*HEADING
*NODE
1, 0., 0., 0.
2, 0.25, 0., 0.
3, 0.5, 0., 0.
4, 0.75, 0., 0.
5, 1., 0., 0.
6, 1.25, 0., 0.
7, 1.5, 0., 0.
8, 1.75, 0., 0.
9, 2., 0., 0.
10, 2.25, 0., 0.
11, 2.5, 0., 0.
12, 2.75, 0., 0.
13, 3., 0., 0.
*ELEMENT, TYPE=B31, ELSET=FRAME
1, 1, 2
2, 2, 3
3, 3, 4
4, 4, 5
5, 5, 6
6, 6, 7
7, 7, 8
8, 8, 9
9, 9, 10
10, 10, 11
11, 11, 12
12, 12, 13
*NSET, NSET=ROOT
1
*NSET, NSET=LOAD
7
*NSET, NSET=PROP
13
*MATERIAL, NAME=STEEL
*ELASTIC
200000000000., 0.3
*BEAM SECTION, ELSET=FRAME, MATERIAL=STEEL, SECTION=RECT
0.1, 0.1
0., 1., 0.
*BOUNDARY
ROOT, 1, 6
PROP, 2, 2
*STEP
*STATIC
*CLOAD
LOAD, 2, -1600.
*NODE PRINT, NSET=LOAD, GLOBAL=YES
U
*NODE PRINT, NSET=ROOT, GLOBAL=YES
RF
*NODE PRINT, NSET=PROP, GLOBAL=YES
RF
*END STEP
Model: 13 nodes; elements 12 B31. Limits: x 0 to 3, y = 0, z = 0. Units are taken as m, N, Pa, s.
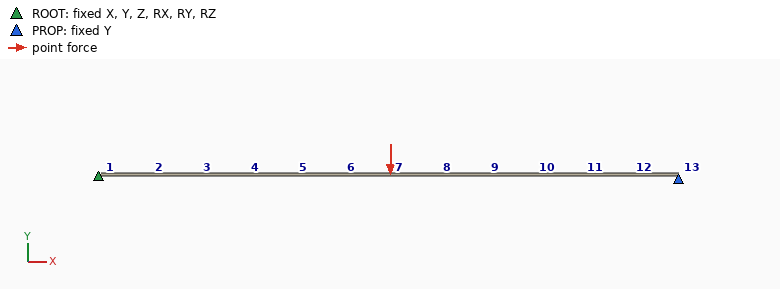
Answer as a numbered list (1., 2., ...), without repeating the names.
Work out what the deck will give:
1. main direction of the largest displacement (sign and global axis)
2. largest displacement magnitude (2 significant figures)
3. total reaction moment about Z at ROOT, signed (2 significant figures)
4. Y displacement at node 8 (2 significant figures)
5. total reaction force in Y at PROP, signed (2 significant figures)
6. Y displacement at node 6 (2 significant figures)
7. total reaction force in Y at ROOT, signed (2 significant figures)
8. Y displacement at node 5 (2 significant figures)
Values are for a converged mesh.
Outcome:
1. -Y
2. 2.4e-04 m
3. 900 N·m
4. -2.4e-04 m
5. 500 N
6. -2.1e-04 m
7. 1100 N
8. -1.6e-04 m
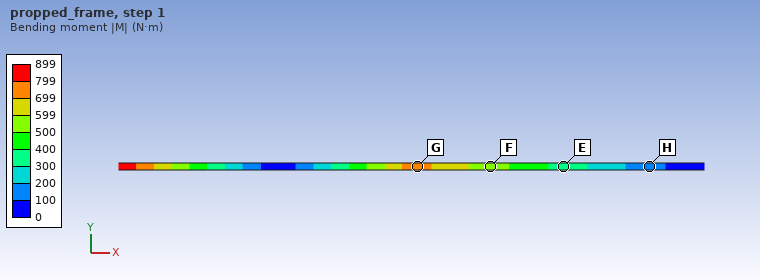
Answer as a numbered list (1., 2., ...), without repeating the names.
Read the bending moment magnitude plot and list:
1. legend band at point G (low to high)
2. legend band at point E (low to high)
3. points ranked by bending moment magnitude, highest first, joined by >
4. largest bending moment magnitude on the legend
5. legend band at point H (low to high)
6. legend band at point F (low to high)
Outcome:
1. 699 to 799 N·m
2. 300 to 400 N·m
3. G > F > E > H
4. 899 N·m
5. 100 to 200 N·m
6. 500 to 599 N·m
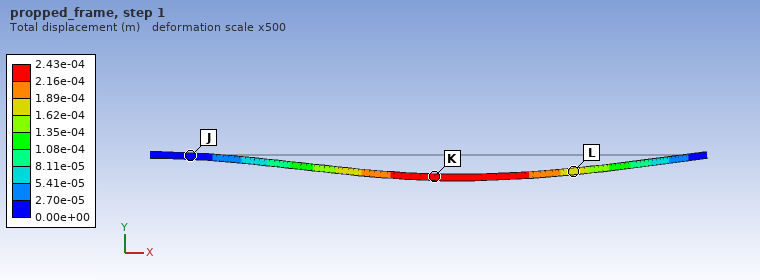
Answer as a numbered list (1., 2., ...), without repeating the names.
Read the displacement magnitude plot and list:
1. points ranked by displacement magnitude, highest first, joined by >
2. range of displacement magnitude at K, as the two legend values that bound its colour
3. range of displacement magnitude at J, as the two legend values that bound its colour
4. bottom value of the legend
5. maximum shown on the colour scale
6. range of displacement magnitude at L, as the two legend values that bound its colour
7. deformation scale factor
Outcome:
1. K > L > J
2. 2.16e-04 to 2.43e-04 m
3. 0.00e+00 to 2.70e-05 m
4. 0.00e+00 m
5. 2.43e-04 m
6. 1.62e-04 to 1.89e-04 m
7. 500
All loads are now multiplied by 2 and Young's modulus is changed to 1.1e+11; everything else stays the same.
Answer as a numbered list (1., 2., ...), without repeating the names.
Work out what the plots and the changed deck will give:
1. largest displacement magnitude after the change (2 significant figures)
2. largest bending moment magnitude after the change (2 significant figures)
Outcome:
1. 8.8e-04 m
2. 1800 N·m
